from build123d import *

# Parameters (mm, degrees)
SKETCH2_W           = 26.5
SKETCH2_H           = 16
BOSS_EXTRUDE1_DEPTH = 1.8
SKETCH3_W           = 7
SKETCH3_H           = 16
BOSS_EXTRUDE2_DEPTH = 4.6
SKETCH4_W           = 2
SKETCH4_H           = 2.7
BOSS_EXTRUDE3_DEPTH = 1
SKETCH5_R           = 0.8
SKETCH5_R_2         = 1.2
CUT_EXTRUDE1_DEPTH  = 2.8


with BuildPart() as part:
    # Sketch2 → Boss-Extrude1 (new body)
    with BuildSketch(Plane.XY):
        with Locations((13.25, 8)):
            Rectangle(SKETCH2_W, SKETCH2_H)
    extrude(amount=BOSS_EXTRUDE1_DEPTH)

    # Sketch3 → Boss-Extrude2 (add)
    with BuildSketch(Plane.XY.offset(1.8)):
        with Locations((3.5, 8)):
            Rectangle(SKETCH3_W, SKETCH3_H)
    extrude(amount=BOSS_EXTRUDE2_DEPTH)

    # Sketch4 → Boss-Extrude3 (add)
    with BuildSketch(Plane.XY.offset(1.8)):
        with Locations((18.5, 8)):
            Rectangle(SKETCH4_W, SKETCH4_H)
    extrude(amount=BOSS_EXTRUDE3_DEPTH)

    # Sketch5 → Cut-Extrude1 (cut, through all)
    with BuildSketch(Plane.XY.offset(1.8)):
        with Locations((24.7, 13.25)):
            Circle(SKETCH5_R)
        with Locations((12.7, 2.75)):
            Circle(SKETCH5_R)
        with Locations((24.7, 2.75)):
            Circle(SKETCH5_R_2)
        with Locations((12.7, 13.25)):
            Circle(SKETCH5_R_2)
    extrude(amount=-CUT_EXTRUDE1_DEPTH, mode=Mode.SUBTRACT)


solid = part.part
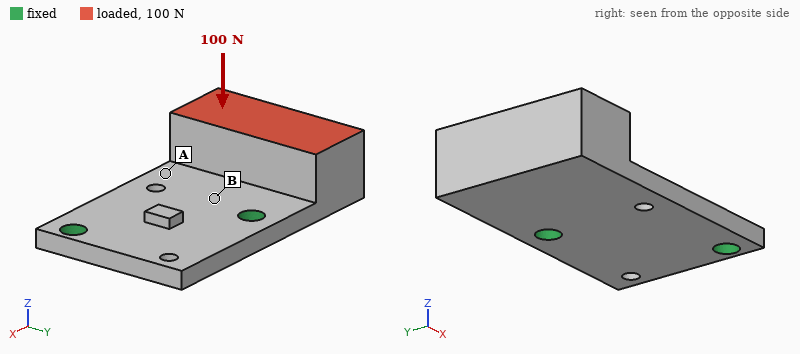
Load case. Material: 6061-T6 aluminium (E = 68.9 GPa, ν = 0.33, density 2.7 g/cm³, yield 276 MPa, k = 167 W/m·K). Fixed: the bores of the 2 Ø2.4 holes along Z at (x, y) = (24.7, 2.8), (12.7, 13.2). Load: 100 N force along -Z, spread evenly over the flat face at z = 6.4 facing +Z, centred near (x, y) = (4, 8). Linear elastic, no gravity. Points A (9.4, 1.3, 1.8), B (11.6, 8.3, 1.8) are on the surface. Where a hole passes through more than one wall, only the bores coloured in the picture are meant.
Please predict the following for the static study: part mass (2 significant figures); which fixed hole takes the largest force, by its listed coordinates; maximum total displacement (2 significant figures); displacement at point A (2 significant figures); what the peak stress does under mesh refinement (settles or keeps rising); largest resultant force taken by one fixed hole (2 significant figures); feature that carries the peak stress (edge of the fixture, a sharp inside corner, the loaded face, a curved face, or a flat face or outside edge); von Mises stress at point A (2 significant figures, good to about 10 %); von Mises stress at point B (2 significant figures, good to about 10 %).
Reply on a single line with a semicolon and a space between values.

3.4 g; (12.7, 13.2); 0.15 mm; 0.053 mm; keeps rising; 110 N; edge of the fixture; 35 MPa; 70 MPa
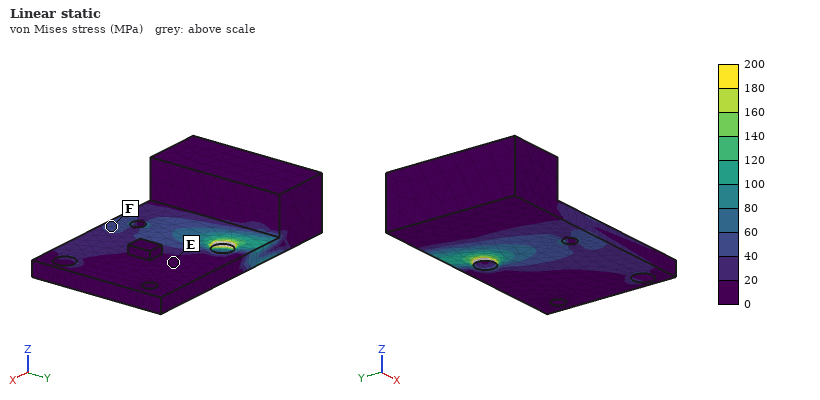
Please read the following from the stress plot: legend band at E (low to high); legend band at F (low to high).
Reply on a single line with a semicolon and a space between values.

0 to 20 MPa; 40 to 60 MPa
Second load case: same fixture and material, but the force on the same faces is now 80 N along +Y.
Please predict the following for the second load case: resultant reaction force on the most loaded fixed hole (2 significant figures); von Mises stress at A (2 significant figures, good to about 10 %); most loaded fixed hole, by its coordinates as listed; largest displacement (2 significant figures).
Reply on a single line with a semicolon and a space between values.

100 N; 22 MPa; (12.7, 13.2); 50 µm
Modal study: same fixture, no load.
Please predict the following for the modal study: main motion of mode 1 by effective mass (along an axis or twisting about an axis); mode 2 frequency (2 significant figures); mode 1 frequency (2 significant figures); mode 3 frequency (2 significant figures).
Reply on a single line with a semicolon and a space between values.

along Z; 8300 Hz; 3600 Hz; 17 kHz
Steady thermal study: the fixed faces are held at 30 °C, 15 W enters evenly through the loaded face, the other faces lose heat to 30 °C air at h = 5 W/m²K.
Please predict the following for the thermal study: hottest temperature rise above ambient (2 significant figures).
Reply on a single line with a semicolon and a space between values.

35 K
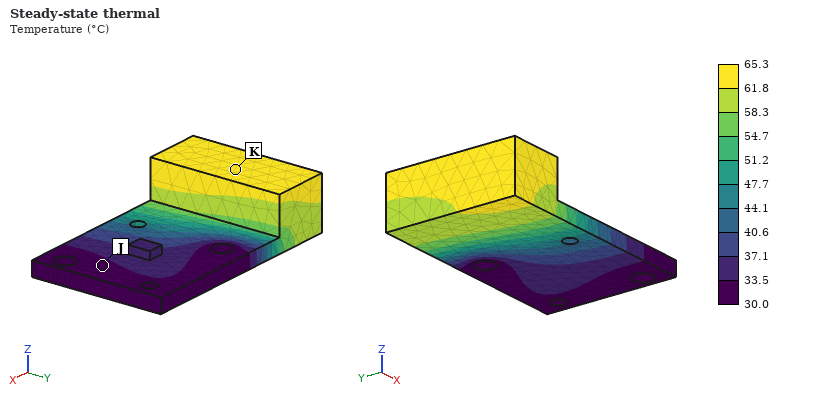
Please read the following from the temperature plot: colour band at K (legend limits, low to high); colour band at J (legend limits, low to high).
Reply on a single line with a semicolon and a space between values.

61.8 to 65.3 °C; 30.0 to 33.5 °C
